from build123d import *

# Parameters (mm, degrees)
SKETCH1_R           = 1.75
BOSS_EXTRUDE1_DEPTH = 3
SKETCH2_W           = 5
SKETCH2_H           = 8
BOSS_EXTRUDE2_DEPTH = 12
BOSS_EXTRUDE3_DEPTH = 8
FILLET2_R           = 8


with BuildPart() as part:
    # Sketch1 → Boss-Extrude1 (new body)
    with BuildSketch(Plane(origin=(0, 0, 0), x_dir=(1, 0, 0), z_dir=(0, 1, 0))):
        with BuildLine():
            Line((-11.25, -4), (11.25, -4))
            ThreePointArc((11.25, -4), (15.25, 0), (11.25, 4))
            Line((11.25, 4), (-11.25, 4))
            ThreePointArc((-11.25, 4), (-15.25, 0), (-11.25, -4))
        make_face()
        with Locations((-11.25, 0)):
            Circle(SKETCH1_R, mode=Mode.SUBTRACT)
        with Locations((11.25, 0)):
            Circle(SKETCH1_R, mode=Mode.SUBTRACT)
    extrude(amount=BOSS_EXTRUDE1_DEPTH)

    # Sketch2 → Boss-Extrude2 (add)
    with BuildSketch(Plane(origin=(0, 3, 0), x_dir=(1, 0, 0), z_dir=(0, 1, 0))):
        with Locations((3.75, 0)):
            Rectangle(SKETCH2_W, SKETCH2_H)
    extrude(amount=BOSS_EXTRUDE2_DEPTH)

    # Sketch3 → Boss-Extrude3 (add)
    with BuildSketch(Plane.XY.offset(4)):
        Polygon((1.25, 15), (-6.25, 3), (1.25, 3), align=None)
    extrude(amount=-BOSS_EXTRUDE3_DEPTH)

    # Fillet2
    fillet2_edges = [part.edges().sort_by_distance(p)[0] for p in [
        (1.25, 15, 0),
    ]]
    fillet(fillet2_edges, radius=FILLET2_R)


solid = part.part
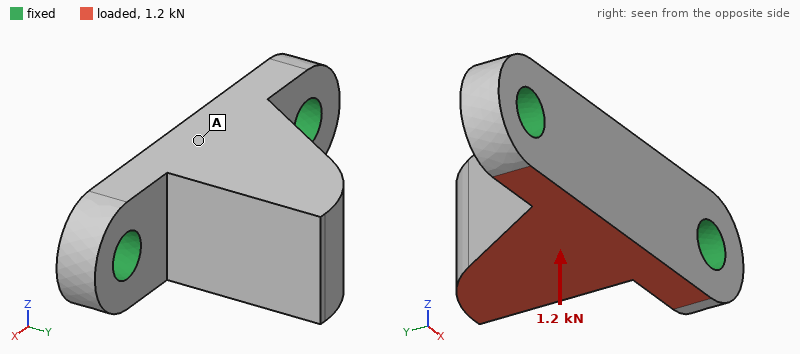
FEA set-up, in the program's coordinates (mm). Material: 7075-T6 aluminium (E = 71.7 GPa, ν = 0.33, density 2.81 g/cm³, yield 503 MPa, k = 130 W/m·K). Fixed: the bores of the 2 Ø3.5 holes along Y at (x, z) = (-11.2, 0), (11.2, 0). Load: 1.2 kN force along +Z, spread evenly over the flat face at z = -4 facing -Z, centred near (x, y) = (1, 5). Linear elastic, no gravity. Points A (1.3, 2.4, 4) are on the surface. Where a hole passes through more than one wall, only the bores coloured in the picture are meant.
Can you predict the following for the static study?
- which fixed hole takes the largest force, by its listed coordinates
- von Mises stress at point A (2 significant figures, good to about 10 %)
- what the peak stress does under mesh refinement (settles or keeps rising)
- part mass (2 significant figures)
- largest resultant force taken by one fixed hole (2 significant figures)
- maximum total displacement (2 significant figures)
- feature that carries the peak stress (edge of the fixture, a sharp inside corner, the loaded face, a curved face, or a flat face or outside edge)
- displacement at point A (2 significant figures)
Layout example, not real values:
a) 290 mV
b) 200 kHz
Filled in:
a) (11.2, 0)
b) 34 MPa
c) keeps rising
d) 4.1 g
e) 660 N
f) 0.10 mm
g) edge of the fixture
h) 0.030 mm
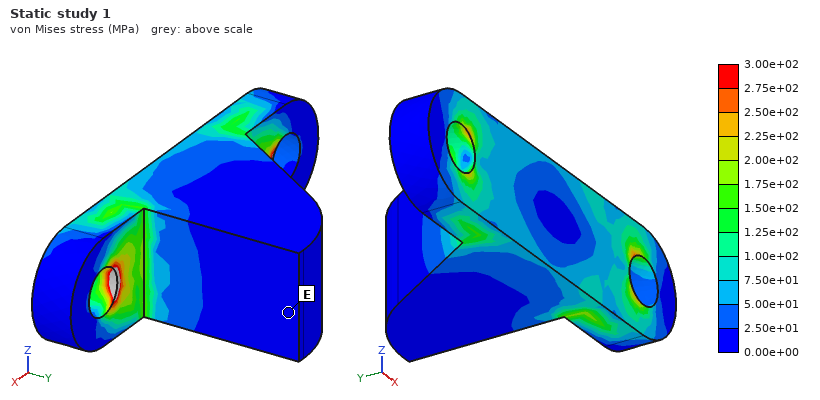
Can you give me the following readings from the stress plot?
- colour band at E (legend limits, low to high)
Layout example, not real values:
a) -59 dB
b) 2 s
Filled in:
a) 0.00e+00 to 2.50e+01 MPa
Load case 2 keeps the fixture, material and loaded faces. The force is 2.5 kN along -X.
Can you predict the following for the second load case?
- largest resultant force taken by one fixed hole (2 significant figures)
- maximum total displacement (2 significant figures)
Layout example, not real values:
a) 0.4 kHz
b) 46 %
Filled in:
a) 1.5 kN
b) 41 µm
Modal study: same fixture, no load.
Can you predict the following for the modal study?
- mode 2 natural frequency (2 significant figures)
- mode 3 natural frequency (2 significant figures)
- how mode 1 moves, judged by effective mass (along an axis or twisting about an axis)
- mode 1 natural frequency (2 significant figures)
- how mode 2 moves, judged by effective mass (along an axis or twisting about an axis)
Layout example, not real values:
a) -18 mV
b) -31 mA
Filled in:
a) 26 kHz
b) 29 kHz
c) along Z
d) 11 kHz
e) along Y
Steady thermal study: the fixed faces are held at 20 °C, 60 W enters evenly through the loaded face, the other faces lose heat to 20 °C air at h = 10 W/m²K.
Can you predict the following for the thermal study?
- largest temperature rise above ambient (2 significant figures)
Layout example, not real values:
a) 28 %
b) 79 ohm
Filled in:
a) 78 K
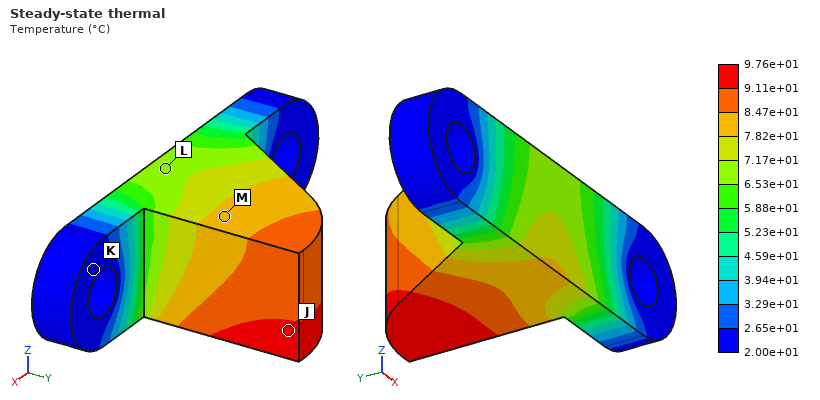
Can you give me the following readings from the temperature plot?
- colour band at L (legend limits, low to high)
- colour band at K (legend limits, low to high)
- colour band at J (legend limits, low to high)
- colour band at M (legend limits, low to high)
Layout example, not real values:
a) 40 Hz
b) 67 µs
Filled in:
a) 6.53e+01 to 7.17e+01 °C
b) 2.00e+01 to 2.65e+01 °C
c) 9.11e+01 to 9.76e+01 °C
d) 7.82e+01 to 8.47e+01 °C
